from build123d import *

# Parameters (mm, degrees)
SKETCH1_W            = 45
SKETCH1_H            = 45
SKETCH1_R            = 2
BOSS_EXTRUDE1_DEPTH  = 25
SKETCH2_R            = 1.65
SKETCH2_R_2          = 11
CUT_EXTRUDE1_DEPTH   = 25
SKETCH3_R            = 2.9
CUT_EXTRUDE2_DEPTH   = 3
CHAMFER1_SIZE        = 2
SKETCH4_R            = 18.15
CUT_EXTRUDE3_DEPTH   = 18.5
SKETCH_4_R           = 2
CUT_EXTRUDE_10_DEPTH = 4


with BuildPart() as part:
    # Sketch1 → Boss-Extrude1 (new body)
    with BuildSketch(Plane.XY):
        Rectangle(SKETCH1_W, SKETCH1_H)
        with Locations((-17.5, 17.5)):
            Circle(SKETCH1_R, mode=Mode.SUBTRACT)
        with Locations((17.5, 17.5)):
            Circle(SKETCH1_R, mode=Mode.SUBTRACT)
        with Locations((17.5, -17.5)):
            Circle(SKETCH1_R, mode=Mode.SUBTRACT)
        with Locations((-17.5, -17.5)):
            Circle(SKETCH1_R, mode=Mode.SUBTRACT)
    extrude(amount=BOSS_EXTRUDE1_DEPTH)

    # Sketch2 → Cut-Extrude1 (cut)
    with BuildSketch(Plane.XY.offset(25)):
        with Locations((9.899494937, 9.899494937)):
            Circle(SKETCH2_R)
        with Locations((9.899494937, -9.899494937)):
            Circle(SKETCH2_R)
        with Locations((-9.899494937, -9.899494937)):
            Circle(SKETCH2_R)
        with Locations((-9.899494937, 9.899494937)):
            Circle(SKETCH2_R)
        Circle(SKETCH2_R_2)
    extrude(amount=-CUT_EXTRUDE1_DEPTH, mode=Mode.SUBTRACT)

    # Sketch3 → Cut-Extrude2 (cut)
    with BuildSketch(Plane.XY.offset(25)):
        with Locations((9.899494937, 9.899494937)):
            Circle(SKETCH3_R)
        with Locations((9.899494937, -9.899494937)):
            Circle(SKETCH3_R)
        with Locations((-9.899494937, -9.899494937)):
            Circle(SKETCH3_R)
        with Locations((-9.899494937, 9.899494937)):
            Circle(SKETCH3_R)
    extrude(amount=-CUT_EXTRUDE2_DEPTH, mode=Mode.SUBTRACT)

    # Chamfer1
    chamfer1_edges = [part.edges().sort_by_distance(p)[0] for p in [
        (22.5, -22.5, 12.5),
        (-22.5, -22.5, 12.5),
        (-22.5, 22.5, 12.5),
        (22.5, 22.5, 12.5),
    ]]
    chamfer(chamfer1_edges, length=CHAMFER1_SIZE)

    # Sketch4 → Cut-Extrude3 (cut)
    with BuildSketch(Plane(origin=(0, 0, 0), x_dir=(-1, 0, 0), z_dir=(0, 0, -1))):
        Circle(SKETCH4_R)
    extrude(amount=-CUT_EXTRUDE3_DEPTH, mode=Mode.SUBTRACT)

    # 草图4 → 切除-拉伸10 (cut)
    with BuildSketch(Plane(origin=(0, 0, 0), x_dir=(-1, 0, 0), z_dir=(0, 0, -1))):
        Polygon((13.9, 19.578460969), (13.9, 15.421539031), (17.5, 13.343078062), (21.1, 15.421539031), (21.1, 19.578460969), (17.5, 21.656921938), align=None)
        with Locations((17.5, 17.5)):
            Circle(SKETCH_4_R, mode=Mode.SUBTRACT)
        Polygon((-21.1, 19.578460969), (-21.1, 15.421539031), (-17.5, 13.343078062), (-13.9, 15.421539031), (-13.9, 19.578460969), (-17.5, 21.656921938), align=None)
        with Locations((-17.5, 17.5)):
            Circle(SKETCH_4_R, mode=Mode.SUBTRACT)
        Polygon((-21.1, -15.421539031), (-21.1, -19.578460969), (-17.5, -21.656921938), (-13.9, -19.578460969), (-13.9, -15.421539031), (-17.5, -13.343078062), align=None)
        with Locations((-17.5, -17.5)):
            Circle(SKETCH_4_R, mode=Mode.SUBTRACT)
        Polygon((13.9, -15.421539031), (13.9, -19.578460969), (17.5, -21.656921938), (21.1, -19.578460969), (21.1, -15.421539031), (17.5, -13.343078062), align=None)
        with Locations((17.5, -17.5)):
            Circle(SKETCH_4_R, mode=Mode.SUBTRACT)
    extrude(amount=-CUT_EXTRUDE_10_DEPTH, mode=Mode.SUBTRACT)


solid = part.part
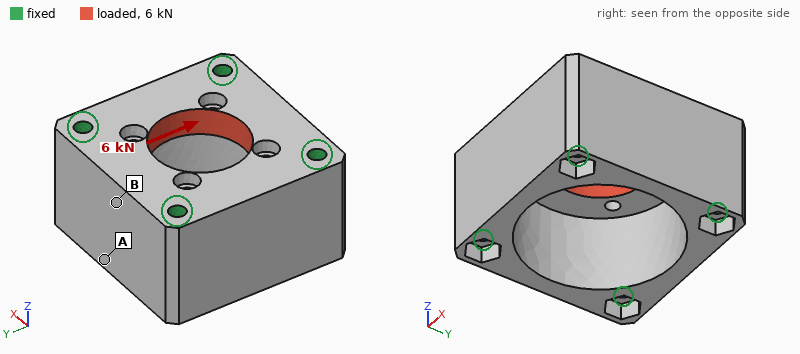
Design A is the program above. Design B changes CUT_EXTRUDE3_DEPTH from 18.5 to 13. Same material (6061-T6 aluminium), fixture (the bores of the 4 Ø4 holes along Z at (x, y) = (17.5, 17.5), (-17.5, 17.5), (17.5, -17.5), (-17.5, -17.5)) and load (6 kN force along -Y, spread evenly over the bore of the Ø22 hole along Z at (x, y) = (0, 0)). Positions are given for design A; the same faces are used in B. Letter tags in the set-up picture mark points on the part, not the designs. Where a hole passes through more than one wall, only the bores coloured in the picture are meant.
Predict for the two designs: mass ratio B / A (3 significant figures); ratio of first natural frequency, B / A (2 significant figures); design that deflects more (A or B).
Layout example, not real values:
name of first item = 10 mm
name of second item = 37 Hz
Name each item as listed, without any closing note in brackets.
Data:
mass ratio B / A = 1.13
ratio of first natural frequency, B / A = 1.0
design that deflects more = A
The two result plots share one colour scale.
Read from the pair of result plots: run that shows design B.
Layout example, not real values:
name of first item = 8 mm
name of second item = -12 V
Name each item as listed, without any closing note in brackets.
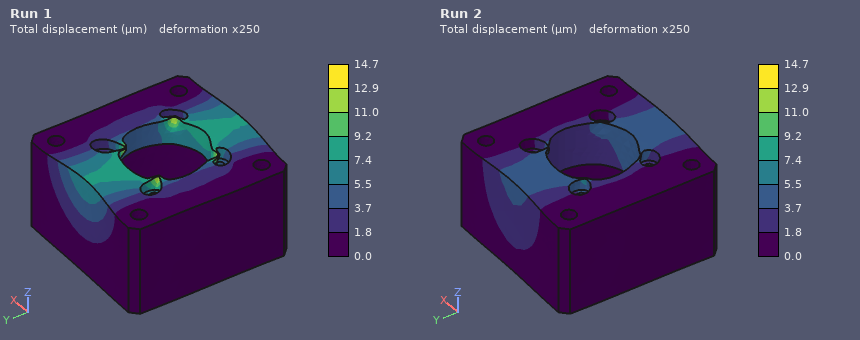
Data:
run that shows design B = Run 2
